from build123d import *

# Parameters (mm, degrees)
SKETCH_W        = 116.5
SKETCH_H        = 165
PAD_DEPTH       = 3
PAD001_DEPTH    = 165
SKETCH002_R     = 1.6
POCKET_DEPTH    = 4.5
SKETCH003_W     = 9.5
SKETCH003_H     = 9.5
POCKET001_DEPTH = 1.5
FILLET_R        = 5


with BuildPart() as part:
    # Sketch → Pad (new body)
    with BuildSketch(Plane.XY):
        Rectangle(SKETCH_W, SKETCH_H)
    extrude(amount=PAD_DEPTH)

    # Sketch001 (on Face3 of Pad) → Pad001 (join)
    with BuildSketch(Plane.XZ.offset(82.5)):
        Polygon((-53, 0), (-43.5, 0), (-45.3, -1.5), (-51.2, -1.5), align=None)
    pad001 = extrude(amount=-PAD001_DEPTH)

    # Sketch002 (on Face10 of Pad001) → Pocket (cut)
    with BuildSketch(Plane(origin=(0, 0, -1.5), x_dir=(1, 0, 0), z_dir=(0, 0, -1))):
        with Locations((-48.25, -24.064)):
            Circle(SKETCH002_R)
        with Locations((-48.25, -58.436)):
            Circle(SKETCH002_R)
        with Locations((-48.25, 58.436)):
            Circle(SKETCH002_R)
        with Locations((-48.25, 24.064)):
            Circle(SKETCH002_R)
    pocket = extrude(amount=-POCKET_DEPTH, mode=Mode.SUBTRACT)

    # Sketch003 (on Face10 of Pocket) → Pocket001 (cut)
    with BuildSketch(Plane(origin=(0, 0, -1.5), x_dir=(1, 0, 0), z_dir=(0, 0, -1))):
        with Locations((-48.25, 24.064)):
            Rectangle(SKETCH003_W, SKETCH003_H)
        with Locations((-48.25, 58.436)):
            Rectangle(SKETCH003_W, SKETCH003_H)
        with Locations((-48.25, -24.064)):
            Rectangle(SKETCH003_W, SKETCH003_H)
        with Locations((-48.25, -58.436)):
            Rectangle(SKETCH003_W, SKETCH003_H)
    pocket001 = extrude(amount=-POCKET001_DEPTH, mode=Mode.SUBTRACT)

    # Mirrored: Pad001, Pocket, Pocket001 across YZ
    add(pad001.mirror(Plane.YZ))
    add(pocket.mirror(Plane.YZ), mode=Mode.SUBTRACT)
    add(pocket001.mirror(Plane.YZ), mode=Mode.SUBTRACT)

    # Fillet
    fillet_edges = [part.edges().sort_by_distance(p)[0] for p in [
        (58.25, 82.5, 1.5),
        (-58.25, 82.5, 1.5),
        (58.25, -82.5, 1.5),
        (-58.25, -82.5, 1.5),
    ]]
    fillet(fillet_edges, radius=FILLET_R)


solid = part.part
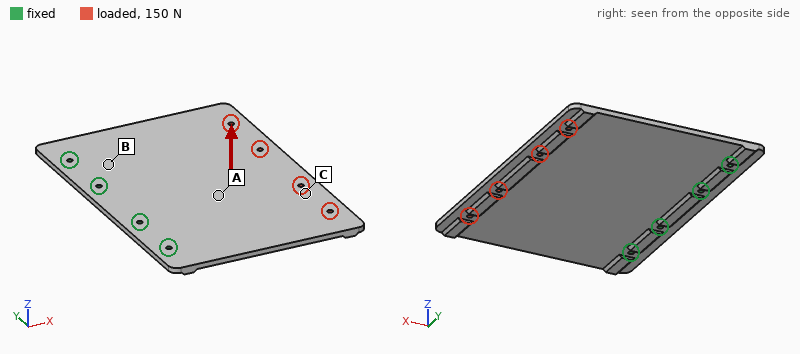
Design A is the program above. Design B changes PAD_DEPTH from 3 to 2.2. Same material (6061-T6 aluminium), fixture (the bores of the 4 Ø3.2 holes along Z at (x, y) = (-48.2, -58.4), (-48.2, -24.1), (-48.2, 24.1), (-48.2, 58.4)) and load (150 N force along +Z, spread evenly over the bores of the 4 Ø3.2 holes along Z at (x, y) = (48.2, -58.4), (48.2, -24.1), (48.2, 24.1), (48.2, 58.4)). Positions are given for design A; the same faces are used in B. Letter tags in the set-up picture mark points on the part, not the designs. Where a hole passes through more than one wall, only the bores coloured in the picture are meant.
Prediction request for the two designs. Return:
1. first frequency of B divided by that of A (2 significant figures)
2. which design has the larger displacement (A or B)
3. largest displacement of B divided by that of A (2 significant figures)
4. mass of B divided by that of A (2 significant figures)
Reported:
0.74
B
2.4
0.75
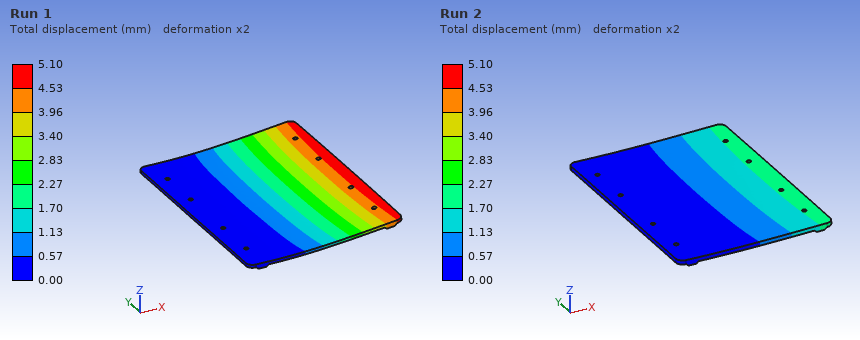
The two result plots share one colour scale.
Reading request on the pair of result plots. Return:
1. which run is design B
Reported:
Run 1
